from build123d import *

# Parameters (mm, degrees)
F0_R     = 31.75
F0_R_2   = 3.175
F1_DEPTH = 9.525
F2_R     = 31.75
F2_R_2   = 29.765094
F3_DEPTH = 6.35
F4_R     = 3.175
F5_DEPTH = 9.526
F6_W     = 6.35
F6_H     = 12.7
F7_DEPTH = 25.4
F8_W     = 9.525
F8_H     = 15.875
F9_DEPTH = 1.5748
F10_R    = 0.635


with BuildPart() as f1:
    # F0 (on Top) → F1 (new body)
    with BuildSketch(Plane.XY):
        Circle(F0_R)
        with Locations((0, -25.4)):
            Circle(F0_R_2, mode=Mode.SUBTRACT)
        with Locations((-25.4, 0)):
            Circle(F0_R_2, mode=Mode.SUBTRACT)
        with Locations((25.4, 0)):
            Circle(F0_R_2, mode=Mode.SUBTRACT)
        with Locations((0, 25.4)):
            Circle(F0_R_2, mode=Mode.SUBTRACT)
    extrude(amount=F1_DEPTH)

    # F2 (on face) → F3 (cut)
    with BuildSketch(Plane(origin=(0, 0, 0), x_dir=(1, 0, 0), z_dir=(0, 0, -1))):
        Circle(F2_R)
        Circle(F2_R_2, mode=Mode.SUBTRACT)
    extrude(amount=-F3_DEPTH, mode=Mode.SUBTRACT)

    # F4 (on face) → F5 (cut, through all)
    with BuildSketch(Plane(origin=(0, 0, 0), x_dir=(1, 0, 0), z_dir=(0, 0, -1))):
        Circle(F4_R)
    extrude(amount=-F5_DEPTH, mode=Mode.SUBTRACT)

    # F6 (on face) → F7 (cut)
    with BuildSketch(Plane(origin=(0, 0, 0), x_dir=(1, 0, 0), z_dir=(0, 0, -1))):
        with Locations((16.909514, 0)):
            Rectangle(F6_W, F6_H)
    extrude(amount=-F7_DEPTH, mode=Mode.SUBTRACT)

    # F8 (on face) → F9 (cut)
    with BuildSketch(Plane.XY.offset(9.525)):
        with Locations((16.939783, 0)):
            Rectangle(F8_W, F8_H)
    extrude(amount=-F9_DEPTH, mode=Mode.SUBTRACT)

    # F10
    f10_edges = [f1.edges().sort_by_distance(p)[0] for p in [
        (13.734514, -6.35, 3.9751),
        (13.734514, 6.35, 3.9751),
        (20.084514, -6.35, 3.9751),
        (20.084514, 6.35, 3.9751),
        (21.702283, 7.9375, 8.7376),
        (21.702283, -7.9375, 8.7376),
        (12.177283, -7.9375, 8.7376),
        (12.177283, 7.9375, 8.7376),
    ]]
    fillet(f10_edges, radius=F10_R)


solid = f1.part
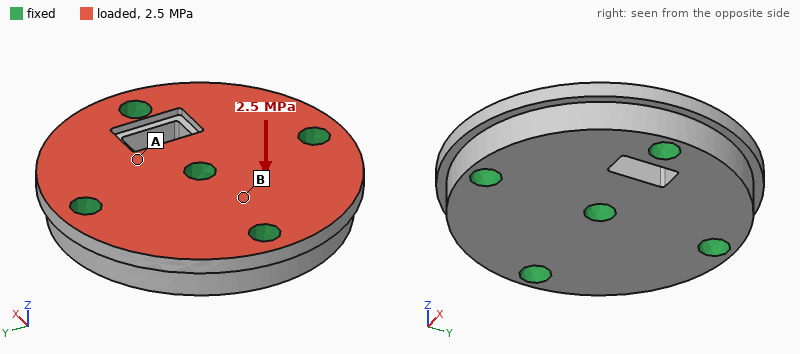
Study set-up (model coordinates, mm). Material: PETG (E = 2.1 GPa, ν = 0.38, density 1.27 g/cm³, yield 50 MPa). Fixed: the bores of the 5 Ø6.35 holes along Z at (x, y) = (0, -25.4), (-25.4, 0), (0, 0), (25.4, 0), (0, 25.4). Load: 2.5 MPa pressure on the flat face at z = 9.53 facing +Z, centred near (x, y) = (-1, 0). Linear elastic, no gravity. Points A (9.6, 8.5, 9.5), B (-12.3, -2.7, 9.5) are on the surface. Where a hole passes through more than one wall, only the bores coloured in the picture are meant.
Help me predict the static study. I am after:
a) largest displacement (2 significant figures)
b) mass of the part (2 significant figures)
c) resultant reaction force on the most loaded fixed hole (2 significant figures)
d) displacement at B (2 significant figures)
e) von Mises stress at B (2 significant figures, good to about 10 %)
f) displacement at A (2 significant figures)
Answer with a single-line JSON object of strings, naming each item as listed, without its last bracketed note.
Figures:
{"largest displacement": "0.26 mm", "mass of the part": "32 g", "resultant reaction force on the most loaded fixed hole": "1.5 kN", "displacement at B": "0.057 mm", "von Mises stress at B": "7.1 MPa", "displacement at A": "0.078 mm"}
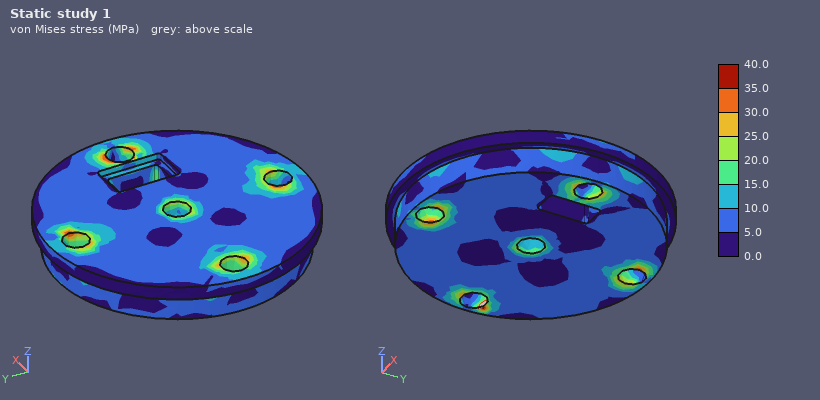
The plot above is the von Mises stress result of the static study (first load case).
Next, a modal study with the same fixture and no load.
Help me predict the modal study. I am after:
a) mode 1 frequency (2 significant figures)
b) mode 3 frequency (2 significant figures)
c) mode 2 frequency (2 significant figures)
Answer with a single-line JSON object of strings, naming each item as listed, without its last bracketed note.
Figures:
{"mode 1 frequency": "6500 Hz", "mode 3 frequency": "6800 Hz", "mode 2 frequency": "6600 Hz"}
